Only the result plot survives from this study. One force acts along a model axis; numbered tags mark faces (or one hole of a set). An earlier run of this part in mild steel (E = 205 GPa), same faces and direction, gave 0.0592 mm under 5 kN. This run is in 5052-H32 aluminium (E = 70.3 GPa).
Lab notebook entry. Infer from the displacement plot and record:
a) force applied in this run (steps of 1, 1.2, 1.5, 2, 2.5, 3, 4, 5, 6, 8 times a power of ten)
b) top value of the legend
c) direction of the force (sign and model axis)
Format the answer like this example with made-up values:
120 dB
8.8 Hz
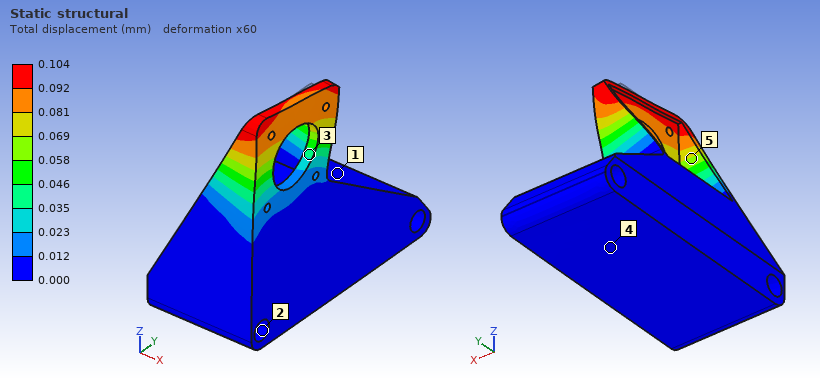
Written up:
3 kN
0.104 mm
+Y
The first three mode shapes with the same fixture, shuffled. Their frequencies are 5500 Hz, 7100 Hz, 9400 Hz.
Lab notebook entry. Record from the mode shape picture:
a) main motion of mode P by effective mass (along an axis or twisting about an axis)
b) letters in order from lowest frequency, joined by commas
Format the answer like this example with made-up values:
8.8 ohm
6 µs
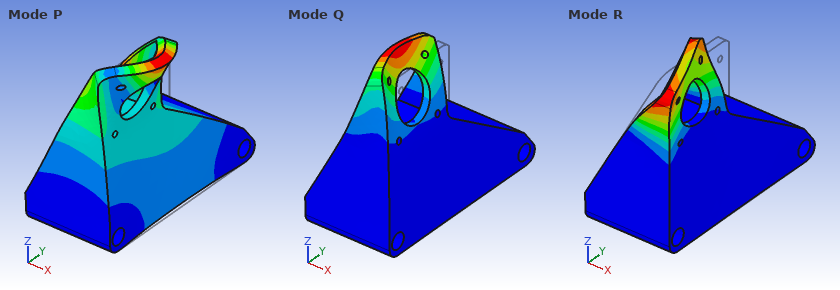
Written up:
along X
Q, R, P
